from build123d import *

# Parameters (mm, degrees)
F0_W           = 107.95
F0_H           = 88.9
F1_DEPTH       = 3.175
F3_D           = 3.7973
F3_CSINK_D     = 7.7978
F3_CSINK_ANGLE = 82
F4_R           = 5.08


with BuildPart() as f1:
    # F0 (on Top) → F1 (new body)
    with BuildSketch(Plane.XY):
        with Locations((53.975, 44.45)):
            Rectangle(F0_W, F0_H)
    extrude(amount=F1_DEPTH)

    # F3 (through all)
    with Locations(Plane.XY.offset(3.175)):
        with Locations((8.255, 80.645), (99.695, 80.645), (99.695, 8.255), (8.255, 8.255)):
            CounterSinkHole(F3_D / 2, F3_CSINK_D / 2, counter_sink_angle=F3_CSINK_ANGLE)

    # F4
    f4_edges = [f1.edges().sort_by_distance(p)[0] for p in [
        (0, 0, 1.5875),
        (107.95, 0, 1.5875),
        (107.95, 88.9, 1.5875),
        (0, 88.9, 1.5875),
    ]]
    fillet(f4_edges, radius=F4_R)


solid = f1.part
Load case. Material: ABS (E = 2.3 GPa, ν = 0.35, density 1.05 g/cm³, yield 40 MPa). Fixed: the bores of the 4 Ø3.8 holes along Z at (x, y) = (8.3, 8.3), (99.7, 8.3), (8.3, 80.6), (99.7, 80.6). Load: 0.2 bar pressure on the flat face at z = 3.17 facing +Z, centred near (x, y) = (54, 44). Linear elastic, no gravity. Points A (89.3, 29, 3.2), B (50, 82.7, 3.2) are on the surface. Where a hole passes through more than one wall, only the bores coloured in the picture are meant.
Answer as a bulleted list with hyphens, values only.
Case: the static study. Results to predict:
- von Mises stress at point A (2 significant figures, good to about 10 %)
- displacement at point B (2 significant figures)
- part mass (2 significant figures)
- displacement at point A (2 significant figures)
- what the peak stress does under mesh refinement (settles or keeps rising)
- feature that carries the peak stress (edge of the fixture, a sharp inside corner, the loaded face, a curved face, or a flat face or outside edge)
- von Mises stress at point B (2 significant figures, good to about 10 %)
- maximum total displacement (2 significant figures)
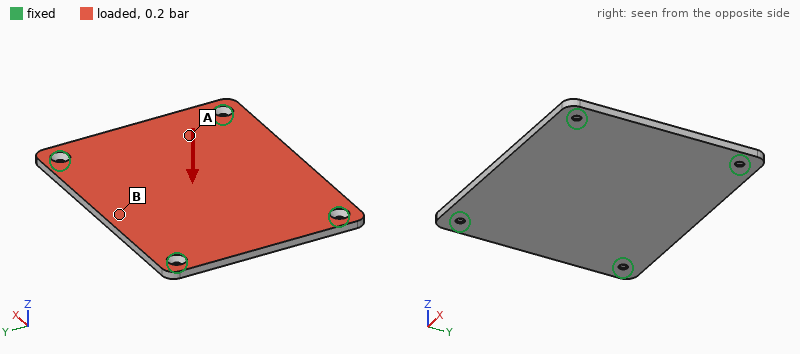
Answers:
- 3.7 MPa
- 1.2 mm
- 32 g
- 0.70 mm
- keeps rising
- edge of the fixture
- 7.3 MPa
- 1.5 mm
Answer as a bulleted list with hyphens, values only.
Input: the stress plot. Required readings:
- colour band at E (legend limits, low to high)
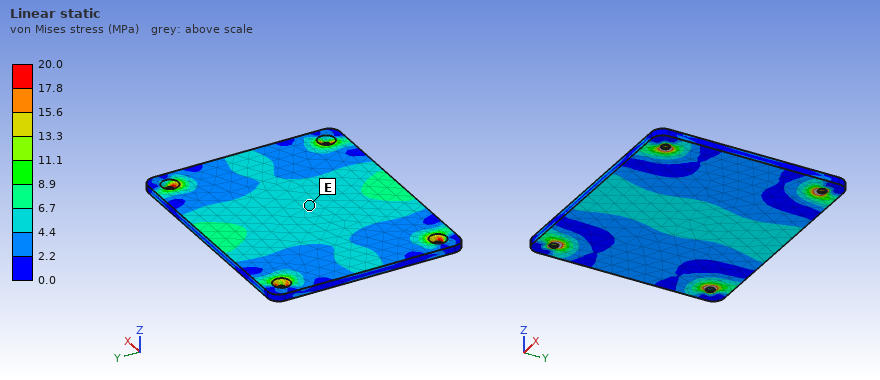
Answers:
- 4.4 to 6.7 MPa
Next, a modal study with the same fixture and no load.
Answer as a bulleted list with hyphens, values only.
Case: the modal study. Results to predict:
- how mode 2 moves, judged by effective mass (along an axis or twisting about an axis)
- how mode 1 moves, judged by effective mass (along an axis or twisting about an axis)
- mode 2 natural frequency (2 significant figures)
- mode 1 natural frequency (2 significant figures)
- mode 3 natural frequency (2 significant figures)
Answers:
- twisting about X
- along Z
- 590 Hz
- 380 Hz
- 750 Hz
